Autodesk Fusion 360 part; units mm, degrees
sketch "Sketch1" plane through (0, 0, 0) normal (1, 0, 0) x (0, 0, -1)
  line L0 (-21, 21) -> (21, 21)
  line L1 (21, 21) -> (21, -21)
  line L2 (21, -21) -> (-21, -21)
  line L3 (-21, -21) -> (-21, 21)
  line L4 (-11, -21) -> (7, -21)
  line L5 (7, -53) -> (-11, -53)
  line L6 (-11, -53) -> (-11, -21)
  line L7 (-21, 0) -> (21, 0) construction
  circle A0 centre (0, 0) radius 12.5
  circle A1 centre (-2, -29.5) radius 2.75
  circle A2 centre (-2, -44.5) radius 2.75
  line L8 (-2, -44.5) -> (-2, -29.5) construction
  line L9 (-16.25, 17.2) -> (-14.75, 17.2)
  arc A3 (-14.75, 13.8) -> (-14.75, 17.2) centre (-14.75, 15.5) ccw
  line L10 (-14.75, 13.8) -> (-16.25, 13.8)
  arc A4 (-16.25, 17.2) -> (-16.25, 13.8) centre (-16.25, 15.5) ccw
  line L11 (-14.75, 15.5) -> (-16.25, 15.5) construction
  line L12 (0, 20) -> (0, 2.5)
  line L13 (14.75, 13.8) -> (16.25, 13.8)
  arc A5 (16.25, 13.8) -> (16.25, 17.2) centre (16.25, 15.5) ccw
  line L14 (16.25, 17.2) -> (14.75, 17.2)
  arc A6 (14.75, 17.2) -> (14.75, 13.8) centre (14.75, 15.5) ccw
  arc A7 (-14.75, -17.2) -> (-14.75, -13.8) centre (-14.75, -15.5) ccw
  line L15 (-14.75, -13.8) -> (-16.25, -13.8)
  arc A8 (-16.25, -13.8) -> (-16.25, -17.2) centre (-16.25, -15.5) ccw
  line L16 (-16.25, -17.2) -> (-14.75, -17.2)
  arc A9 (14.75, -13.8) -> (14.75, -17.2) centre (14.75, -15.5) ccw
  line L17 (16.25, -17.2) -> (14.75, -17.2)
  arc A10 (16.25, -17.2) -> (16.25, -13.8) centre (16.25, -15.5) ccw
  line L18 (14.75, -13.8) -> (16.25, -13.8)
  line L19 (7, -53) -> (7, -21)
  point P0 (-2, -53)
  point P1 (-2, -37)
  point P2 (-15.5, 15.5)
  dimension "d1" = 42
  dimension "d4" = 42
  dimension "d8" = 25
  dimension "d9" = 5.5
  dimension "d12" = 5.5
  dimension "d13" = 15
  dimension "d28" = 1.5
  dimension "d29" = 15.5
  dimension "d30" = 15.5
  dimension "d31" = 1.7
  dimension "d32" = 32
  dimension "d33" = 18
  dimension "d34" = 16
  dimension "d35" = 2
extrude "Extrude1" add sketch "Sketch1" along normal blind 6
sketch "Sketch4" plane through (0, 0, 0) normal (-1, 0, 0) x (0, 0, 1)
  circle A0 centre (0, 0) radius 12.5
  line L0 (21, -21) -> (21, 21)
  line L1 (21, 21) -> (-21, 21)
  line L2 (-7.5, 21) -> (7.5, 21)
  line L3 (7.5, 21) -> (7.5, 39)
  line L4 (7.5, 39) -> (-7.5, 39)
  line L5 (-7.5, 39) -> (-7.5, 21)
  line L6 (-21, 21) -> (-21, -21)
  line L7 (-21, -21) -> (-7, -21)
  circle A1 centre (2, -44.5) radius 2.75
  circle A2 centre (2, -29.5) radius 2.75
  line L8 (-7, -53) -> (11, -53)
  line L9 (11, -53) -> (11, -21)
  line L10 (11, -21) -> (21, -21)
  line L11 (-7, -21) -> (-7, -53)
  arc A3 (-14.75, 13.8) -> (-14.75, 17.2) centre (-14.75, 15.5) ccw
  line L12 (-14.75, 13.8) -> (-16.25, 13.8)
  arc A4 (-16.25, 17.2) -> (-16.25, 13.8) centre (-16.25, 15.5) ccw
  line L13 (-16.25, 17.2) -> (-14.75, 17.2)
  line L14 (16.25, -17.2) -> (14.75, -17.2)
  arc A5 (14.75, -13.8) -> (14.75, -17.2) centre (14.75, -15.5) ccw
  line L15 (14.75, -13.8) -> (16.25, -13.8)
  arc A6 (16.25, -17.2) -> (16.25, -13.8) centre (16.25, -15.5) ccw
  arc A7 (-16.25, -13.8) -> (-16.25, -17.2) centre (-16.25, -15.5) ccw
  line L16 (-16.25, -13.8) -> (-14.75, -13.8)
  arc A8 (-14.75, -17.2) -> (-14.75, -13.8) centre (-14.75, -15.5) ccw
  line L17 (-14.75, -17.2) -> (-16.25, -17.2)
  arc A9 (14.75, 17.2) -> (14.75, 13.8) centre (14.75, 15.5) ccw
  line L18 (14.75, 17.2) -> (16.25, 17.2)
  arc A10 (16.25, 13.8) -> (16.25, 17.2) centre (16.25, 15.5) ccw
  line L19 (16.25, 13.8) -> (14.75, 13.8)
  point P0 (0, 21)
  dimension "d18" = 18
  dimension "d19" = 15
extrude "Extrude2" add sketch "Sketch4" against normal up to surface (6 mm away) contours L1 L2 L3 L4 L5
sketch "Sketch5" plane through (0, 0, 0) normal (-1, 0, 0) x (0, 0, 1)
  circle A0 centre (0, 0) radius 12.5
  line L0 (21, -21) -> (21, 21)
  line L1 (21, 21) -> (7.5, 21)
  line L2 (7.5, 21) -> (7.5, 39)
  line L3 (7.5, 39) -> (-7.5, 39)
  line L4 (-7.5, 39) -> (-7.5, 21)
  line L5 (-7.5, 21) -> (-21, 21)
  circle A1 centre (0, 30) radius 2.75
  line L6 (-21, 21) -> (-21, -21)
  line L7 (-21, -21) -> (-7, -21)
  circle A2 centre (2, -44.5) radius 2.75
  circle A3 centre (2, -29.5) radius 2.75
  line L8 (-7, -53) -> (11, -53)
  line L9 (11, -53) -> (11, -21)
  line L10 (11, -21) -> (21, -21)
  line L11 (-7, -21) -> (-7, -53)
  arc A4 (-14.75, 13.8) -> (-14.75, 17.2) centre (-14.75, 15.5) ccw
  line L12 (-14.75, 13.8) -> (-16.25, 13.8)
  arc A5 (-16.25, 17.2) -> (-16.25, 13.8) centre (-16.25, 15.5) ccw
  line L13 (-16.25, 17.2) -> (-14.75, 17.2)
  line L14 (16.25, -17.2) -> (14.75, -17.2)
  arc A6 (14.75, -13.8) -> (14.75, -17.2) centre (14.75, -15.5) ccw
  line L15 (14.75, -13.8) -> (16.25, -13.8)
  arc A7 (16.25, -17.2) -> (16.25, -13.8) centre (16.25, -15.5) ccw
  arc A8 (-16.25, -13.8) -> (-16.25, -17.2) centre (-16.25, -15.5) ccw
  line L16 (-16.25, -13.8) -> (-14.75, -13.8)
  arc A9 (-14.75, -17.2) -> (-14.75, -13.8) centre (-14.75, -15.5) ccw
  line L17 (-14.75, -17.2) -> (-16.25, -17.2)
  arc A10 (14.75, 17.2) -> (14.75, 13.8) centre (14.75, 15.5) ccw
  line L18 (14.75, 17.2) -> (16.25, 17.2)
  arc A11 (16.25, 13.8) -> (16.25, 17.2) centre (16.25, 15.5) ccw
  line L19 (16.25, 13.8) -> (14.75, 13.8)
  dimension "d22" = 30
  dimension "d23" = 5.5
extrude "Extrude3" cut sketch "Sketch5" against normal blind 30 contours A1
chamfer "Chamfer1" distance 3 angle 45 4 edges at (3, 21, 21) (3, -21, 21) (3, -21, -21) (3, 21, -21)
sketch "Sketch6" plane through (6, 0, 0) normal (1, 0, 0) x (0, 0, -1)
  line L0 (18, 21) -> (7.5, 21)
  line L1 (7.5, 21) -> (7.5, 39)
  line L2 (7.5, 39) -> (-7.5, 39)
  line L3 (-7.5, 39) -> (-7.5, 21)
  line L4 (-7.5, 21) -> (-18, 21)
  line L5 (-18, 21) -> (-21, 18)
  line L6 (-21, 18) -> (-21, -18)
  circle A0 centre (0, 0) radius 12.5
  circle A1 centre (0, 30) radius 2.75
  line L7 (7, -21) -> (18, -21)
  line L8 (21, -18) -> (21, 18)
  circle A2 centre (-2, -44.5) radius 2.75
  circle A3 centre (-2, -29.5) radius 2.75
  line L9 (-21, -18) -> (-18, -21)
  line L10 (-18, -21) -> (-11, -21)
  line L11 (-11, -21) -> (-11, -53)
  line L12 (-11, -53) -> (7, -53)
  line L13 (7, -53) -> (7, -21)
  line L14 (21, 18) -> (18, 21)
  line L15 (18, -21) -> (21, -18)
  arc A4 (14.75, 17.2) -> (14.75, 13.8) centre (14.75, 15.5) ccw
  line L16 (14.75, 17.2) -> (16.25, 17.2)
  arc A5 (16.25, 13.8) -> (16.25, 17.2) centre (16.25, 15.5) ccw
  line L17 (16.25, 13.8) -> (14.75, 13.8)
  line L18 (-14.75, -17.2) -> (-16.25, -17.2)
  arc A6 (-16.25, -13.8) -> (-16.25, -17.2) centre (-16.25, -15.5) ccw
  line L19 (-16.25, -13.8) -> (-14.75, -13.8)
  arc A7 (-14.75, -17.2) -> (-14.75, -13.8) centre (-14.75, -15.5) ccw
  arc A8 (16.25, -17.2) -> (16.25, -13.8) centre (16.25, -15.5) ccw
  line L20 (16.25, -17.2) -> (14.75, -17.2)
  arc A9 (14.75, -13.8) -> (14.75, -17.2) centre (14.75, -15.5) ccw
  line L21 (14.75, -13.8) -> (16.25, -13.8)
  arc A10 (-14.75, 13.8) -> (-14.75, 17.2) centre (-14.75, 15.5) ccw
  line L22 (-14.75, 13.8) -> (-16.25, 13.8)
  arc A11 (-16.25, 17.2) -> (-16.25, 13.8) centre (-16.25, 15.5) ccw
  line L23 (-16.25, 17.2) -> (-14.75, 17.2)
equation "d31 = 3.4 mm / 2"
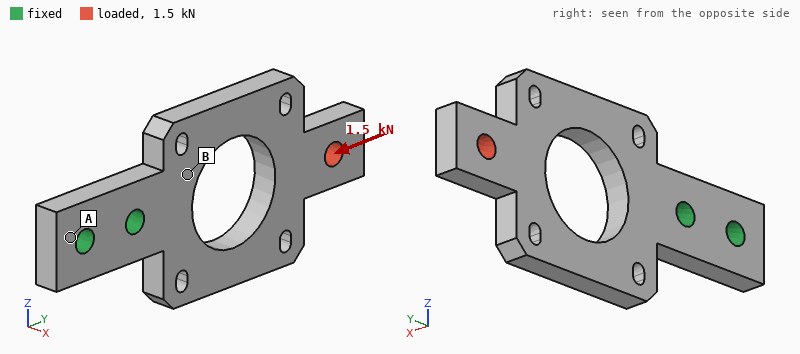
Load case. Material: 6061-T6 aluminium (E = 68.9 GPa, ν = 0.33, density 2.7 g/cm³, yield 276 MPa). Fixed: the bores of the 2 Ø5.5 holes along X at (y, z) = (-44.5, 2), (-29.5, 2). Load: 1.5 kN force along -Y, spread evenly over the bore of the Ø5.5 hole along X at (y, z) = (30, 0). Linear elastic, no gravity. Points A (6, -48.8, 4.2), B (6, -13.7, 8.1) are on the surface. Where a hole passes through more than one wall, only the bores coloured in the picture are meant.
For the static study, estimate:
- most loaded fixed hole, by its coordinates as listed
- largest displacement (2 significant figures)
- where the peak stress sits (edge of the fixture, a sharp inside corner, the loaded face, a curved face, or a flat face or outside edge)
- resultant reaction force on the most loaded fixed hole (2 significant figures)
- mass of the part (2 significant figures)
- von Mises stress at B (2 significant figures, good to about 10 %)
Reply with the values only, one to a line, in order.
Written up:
(-29.5, 2)
56 µm
a curved face
1.3 kN
32 g
20 MPa
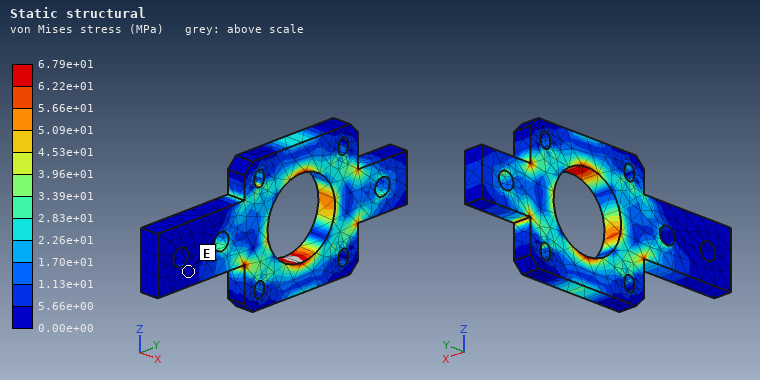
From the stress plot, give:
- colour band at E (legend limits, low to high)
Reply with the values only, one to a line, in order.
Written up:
0.00e+00 to 5.66e+00 MPa
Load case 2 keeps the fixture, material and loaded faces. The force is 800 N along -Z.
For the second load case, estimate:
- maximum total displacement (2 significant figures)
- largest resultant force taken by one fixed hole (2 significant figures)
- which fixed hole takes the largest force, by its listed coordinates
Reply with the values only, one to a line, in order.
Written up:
0.42 mm
2.3 kN
(-29.5, 2)
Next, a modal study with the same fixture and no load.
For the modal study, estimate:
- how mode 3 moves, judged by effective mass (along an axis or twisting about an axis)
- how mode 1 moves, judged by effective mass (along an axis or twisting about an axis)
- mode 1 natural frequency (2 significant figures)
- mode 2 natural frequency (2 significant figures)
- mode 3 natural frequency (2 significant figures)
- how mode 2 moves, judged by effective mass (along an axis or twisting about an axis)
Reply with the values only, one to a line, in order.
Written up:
twisting about Y
along X
1000 Hz
2400 Hz
3000 Hz
along Z
